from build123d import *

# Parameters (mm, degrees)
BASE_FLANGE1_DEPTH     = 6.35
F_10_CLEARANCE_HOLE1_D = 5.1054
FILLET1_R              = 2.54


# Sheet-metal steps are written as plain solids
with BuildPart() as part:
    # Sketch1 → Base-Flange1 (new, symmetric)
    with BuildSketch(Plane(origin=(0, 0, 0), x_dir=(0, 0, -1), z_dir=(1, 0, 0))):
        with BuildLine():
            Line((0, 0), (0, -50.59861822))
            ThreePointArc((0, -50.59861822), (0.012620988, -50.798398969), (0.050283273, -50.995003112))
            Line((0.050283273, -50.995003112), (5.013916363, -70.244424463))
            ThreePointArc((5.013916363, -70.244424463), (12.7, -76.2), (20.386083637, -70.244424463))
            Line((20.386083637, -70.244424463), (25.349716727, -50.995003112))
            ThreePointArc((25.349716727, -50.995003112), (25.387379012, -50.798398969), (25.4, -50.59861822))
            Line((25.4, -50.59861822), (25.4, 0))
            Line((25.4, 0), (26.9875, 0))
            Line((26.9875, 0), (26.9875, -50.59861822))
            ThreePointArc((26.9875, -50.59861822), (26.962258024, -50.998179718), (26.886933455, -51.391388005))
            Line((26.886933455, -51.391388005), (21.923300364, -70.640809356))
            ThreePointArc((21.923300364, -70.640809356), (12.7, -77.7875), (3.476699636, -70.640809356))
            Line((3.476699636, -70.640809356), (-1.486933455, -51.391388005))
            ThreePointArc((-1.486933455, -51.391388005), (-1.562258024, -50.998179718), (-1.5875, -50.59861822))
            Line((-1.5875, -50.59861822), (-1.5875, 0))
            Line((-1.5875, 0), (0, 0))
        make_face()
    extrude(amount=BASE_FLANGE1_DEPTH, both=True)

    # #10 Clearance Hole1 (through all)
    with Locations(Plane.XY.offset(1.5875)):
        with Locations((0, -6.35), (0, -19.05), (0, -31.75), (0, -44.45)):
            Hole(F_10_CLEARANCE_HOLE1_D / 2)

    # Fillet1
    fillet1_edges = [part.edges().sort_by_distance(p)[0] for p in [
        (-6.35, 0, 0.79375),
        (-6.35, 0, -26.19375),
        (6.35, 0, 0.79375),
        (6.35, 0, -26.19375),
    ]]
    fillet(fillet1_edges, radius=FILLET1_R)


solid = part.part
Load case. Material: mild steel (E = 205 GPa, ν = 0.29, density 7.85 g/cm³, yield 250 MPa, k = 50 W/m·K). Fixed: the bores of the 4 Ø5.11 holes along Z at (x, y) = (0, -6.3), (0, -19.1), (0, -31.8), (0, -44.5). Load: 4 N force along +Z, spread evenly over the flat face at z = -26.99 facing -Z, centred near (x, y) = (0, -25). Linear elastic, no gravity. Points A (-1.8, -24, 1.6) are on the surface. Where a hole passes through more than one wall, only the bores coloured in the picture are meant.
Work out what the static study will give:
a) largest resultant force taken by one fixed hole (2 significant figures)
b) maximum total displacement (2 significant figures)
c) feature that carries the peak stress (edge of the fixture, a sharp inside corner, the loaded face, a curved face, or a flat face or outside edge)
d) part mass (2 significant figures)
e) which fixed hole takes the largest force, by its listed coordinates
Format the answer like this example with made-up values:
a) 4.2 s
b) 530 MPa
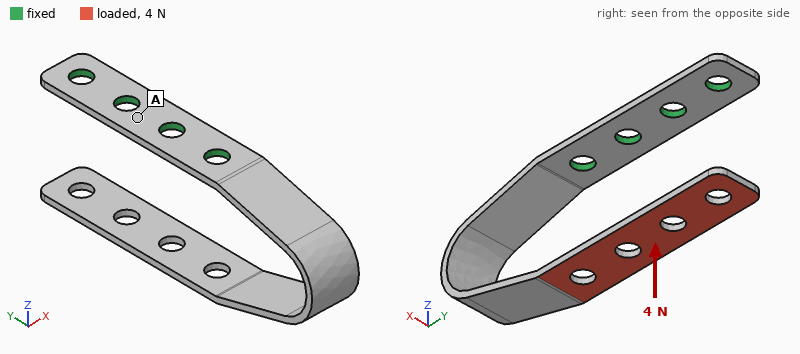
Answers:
a) 4.1 N
b) 0.91 mm
c) a curved face
d) 24 g
e) (0, -44.5)
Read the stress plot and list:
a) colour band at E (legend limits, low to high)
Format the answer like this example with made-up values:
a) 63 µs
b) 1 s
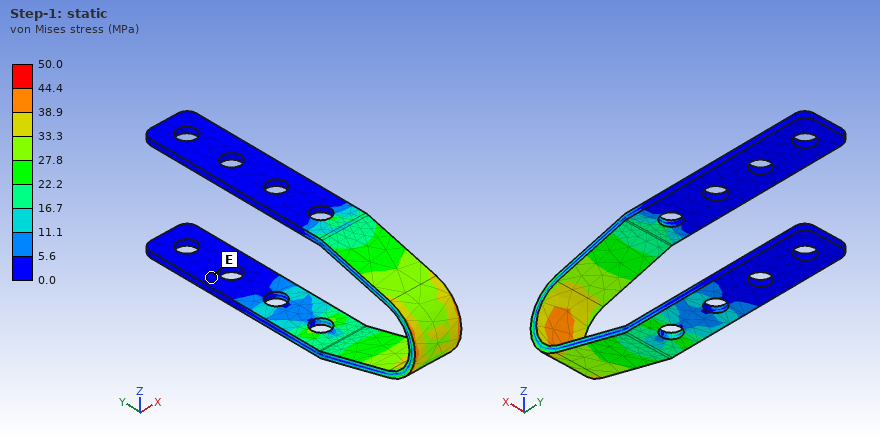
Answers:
a) 0.0 to 5.6 MPa
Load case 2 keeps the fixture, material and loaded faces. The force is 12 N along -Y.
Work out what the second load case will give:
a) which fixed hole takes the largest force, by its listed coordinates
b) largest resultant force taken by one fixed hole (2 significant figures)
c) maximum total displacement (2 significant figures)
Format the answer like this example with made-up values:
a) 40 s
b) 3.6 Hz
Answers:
a) (0, -44.5)
b) 12 N
c) 0.95 mm
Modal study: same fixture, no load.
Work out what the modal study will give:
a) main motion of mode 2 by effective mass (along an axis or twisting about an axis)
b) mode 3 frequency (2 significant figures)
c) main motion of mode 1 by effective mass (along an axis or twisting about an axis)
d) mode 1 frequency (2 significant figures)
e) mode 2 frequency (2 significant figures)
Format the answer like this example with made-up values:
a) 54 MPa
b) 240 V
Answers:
a) along X
b) 450 Hz
c) along Z
d) 140 Hz
e) 240 Hz
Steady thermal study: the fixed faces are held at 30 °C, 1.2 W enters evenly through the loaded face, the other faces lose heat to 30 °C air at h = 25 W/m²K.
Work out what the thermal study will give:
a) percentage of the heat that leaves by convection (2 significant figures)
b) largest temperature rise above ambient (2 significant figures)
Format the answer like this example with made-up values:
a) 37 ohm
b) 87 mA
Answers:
a) 86 %
b) 36 K
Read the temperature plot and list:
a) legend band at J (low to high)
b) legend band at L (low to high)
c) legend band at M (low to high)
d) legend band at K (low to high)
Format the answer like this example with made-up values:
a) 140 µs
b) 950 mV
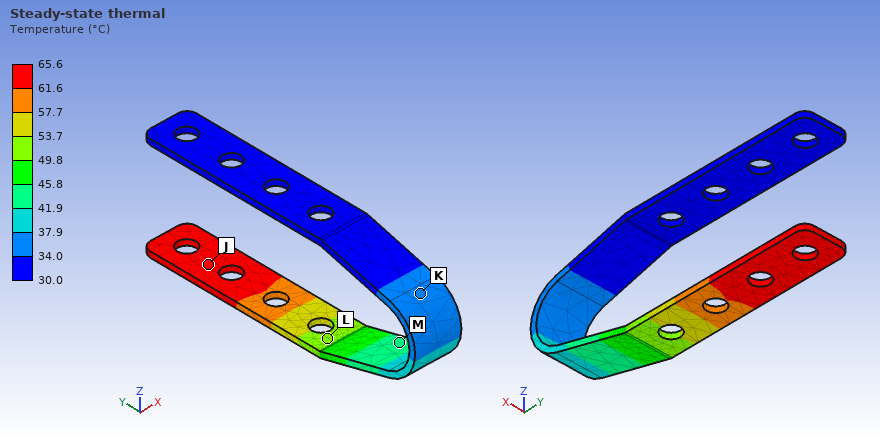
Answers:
a) 61.6 to 65.6 °C
b) 49.8 to 53.7 °C
c) 41.9 to 45.8 °C
d) 34.0 to 37.9 °C
